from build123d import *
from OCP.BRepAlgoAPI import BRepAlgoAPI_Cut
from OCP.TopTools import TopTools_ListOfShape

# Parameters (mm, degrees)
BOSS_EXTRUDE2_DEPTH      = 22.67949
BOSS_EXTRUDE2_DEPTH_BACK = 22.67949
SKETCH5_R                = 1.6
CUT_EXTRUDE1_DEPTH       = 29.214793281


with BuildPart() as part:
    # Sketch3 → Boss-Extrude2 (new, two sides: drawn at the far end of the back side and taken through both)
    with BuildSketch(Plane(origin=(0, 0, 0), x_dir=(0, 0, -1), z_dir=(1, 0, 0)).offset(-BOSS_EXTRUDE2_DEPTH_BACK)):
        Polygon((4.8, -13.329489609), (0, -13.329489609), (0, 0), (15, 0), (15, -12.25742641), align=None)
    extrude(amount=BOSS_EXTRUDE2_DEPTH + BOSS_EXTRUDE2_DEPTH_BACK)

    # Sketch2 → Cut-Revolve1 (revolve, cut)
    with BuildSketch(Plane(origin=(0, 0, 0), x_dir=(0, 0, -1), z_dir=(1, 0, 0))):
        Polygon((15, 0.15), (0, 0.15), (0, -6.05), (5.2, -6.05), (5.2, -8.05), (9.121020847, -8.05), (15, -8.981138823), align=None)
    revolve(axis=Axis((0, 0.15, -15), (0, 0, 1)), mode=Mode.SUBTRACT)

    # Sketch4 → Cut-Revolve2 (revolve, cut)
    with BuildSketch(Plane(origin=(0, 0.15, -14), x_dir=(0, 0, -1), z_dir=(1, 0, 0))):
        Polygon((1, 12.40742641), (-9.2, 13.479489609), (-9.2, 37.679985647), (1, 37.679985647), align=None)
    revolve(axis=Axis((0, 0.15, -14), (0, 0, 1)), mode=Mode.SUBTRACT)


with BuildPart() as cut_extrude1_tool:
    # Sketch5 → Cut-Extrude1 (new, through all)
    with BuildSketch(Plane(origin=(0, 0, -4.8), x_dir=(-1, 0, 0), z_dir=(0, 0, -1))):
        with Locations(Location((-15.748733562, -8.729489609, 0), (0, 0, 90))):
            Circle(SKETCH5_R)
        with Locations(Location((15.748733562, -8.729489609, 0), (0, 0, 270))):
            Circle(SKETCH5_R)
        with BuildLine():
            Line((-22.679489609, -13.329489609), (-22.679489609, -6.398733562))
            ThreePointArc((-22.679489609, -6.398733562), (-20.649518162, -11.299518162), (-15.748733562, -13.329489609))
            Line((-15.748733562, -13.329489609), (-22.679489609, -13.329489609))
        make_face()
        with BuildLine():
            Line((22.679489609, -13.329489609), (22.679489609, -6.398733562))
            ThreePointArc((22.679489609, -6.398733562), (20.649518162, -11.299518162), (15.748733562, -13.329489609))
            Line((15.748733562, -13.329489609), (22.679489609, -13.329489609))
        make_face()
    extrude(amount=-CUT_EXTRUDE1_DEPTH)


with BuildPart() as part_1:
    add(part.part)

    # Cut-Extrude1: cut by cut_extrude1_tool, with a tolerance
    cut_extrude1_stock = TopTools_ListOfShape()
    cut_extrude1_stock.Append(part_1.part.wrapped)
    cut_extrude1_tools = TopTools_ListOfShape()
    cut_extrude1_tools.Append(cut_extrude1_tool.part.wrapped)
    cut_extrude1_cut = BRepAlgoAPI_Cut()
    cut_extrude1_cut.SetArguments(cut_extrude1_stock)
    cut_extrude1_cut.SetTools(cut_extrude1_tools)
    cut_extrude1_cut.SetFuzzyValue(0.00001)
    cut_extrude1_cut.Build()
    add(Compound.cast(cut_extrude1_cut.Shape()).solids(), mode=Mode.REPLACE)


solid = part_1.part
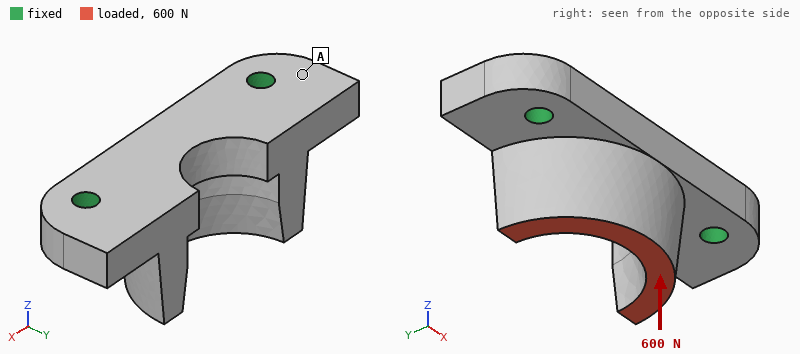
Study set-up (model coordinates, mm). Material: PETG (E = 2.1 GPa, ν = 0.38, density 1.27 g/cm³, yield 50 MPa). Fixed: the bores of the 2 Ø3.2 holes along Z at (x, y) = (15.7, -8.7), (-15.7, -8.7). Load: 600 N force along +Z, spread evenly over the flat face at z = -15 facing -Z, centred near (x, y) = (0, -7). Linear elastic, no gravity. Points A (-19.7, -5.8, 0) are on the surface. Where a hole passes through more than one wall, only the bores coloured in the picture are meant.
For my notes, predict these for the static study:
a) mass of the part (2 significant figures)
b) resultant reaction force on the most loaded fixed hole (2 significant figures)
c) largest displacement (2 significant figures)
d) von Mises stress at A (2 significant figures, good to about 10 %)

5.1 g
320 N
0.19 mm
5.5 MPa
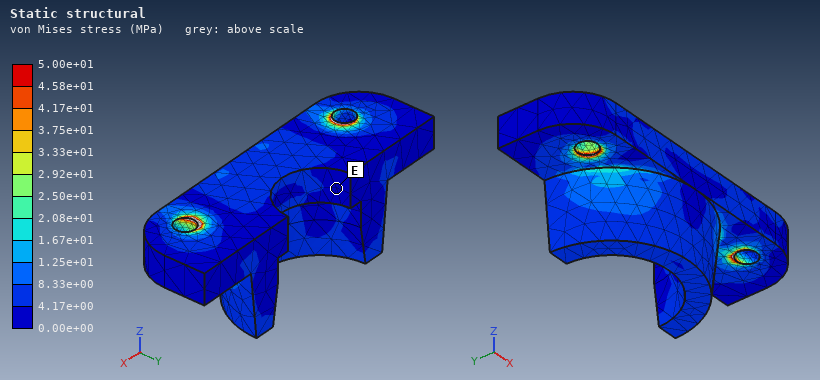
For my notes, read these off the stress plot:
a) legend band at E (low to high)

0.00e+00 to 4.17e+00 MPa
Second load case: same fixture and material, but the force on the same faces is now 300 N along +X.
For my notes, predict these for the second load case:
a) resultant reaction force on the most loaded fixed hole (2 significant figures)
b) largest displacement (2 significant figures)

200 N
0.19 mm
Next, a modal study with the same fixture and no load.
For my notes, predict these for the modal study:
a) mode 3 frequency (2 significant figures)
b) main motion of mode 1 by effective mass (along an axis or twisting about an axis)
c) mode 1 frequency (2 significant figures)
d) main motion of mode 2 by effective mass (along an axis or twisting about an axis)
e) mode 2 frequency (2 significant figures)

6100 Hz
along Y
3400 Hz
along Z
5400 Hz
